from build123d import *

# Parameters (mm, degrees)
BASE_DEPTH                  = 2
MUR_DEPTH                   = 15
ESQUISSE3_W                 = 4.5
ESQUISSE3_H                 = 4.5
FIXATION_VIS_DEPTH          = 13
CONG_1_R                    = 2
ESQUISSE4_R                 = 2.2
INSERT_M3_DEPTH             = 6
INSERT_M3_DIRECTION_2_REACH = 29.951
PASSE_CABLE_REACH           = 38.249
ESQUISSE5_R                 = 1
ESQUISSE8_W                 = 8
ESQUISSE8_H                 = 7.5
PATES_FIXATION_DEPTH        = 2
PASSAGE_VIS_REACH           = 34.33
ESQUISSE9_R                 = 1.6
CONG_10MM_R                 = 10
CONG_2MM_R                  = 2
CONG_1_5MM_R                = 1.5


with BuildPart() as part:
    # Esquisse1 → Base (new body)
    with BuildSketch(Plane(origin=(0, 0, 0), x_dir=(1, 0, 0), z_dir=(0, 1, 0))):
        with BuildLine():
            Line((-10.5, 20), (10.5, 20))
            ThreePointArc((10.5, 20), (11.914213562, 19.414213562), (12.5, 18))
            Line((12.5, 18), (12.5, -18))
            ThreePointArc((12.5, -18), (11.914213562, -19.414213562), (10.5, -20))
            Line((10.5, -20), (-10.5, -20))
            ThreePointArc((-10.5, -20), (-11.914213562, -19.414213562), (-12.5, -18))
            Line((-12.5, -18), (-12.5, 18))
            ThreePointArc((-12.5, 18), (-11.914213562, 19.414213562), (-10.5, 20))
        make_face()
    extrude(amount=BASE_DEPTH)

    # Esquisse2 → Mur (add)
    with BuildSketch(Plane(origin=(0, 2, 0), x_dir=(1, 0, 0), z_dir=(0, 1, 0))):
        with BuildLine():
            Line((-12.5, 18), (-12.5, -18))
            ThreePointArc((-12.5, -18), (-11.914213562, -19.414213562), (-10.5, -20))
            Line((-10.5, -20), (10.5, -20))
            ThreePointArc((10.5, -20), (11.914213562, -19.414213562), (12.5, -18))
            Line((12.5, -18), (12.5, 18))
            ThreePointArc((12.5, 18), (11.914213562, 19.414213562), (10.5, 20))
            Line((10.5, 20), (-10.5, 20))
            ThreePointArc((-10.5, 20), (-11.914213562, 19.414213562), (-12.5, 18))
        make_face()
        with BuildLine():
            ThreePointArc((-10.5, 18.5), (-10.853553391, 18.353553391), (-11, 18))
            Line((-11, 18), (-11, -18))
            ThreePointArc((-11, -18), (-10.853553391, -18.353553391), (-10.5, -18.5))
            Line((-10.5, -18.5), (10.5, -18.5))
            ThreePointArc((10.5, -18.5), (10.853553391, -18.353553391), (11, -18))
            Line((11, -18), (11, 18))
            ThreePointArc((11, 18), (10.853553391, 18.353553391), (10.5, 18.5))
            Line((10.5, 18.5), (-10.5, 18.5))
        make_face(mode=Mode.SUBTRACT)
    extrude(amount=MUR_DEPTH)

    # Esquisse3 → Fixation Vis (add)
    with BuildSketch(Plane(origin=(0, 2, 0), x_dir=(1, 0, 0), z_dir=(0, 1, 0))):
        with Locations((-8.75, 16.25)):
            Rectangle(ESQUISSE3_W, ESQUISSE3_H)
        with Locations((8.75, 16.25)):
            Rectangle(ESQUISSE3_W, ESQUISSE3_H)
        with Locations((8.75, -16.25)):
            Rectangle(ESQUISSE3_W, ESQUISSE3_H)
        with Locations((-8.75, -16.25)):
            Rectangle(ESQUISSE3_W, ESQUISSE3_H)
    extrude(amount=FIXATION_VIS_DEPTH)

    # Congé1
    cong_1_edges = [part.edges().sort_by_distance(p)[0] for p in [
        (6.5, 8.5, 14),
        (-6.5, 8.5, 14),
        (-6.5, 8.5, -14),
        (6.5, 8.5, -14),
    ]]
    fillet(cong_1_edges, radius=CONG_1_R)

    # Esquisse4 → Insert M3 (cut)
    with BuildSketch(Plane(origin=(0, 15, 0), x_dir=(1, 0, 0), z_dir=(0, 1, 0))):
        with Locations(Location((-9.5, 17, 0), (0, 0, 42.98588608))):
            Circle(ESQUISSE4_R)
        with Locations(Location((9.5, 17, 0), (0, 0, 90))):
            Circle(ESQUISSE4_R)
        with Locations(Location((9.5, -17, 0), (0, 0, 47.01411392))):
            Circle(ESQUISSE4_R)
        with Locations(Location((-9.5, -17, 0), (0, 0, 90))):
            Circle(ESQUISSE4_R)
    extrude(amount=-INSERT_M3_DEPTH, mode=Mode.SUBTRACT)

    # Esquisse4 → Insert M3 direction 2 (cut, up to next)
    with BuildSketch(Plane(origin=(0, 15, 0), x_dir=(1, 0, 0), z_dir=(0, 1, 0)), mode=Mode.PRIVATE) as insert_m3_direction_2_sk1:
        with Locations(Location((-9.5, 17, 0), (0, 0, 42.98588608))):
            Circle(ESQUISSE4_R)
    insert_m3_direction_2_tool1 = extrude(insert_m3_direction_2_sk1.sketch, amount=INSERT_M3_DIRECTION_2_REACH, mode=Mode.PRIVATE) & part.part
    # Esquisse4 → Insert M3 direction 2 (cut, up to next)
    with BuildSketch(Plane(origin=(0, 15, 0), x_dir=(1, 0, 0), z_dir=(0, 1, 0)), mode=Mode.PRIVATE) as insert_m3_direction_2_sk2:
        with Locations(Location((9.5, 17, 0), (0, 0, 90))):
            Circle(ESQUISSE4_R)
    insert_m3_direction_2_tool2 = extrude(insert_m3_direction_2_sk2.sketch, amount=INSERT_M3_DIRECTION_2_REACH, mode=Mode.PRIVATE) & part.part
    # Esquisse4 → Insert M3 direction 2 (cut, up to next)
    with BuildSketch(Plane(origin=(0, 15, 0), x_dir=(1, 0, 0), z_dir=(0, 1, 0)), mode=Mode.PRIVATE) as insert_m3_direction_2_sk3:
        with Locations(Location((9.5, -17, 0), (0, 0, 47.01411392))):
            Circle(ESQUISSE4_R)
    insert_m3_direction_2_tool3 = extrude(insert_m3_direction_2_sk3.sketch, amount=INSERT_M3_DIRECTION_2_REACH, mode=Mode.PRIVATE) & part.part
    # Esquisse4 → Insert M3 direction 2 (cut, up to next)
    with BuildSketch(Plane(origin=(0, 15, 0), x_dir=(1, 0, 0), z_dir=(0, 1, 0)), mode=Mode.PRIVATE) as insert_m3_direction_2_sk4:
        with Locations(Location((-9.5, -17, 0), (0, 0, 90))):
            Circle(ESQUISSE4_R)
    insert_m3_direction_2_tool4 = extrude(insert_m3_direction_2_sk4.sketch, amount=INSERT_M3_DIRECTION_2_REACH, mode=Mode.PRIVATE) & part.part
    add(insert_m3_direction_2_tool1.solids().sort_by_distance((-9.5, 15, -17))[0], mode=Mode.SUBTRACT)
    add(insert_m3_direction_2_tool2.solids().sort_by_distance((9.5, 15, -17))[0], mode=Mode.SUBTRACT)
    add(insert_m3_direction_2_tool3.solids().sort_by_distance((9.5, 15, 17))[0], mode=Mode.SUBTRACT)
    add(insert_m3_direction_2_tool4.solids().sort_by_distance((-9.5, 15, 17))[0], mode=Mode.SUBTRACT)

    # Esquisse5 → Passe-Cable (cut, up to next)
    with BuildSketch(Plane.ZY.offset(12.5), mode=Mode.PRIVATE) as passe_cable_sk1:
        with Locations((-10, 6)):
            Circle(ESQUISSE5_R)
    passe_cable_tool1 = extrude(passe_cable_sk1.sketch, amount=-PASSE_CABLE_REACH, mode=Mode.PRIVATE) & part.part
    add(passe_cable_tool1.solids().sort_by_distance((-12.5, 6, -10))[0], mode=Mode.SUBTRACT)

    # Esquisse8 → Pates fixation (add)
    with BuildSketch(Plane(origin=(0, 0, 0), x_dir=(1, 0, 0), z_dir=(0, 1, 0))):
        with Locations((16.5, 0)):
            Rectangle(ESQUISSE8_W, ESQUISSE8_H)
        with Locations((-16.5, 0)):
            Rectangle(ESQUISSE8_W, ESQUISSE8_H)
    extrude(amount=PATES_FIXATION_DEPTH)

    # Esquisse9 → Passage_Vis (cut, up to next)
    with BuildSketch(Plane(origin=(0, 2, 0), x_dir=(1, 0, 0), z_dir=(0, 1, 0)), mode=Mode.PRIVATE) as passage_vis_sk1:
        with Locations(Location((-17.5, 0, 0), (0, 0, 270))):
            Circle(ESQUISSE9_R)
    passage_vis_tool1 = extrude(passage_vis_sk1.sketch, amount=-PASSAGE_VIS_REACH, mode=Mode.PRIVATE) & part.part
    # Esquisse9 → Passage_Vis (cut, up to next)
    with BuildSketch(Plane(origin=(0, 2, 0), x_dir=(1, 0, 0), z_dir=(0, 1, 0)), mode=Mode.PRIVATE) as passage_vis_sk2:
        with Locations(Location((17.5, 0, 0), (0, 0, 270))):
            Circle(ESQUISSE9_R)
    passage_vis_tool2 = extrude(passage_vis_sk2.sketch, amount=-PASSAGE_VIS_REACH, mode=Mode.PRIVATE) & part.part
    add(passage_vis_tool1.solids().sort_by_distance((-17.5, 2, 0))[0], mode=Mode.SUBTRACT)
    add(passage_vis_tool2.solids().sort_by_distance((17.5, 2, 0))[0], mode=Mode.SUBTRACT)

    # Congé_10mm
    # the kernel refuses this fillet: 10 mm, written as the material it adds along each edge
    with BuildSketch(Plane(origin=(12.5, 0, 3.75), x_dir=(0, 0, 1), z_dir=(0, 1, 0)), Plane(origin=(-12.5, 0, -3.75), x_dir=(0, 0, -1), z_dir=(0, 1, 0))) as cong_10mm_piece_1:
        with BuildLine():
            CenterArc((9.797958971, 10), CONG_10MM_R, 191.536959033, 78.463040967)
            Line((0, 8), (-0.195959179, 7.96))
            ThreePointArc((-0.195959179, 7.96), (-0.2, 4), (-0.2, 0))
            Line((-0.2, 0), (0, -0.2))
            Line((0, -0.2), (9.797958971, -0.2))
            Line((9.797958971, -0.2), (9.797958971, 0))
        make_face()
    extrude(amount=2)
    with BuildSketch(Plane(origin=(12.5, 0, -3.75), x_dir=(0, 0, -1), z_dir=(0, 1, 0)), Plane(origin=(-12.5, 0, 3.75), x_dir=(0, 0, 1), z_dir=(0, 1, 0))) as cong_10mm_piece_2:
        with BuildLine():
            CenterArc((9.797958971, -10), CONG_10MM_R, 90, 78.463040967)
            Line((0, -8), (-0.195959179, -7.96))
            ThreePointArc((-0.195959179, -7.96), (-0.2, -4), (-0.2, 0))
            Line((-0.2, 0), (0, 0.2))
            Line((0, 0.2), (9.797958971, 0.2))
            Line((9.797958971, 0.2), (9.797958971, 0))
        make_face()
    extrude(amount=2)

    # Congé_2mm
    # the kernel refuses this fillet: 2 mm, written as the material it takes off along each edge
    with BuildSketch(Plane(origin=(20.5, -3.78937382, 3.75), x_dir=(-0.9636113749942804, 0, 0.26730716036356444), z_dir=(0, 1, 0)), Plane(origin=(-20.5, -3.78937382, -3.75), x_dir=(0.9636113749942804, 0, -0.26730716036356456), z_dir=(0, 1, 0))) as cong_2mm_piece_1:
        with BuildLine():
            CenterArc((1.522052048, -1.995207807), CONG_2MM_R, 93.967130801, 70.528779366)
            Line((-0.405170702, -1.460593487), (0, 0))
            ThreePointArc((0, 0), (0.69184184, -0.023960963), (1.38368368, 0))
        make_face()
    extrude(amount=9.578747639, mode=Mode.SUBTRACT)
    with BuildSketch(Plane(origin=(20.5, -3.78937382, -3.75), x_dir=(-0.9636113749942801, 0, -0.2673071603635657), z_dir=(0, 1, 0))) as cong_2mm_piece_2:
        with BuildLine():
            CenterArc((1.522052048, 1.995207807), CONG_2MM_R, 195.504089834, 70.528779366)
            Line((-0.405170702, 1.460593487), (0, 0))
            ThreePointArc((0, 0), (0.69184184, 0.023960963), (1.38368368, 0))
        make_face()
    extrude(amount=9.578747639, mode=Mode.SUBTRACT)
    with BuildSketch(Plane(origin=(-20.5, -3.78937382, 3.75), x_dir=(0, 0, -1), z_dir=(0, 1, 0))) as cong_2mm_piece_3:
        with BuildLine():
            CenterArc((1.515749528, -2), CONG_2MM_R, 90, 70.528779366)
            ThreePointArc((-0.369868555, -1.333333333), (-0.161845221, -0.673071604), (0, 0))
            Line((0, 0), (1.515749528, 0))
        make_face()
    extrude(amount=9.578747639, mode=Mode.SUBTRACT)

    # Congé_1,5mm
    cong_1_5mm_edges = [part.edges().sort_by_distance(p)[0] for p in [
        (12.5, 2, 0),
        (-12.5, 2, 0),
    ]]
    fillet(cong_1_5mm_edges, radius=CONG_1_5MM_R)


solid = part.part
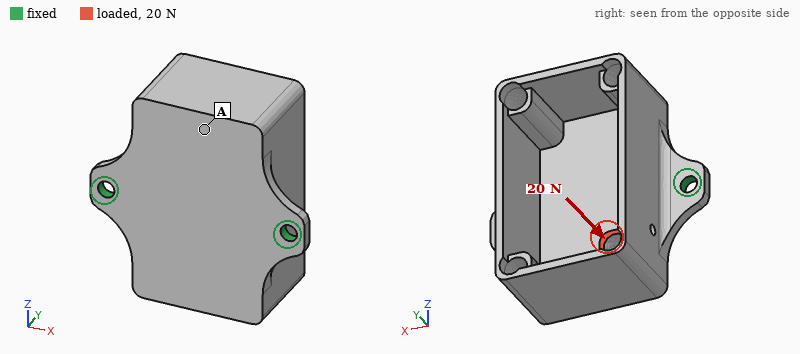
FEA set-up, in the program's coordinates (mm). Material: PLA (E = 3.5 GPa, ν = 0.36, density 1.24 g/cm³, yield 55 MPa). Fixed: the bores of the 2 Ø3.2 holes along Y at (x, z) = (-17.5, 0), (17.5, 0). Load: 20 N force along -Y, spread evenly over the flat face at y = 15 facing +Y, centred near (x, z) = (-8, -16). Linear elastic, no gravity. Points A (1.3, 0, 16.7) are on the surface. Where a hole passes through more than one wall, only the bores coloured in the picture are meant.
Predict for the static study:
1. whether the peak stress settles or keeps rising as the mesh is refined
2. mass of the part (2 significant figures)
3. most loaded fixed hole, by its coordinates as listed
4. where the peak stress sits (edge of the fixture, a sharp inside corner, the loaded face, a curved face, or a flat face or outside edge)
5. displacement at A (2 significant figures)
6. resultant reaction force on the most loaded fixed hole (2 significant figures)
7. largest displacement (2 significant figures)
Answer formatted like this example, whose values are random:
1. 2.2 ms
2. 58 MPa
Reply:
1. keeps rising
2. 7.1 g
3. (-17.5, 0)
4. edge of the fixture
5. 0.18 mm
6. 16 N
7. 0.35 mm
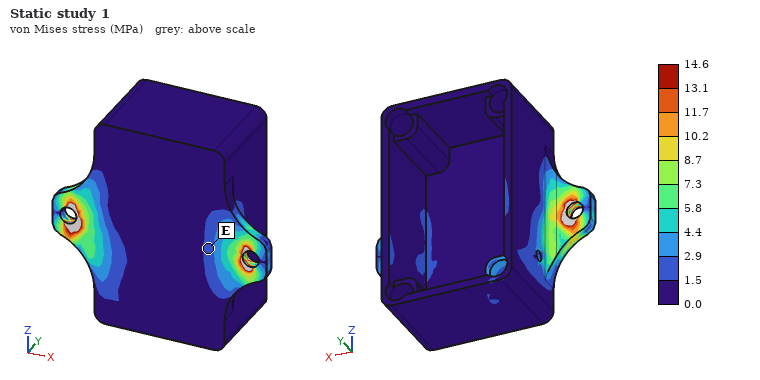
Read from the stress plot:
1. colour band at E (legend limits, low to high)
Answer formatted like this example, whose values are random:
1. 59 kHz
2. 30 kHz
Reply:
1. 1.5 to 2.9 MPa
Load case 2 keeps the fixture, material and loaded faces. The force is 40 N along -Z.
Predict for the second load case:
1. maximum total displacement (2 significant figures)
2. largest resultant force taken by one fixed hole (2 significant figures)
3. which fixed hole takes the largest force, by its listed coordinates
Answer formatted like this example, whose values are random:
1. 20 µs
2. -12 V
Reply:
1. 0.68 mm
2. 30 N
3. (-17.5, 0)
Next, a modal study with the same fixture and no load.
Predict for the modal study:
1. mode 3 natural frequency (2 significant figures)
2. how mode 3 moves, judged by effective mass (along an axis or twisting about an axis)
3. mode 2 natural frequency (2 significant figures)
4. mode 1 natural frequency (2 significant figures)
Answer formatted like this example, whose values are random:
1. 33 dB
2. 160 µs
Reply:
1. 2200 Hz
2. along Y
3. 1700 Hz
4. 650 Hz
